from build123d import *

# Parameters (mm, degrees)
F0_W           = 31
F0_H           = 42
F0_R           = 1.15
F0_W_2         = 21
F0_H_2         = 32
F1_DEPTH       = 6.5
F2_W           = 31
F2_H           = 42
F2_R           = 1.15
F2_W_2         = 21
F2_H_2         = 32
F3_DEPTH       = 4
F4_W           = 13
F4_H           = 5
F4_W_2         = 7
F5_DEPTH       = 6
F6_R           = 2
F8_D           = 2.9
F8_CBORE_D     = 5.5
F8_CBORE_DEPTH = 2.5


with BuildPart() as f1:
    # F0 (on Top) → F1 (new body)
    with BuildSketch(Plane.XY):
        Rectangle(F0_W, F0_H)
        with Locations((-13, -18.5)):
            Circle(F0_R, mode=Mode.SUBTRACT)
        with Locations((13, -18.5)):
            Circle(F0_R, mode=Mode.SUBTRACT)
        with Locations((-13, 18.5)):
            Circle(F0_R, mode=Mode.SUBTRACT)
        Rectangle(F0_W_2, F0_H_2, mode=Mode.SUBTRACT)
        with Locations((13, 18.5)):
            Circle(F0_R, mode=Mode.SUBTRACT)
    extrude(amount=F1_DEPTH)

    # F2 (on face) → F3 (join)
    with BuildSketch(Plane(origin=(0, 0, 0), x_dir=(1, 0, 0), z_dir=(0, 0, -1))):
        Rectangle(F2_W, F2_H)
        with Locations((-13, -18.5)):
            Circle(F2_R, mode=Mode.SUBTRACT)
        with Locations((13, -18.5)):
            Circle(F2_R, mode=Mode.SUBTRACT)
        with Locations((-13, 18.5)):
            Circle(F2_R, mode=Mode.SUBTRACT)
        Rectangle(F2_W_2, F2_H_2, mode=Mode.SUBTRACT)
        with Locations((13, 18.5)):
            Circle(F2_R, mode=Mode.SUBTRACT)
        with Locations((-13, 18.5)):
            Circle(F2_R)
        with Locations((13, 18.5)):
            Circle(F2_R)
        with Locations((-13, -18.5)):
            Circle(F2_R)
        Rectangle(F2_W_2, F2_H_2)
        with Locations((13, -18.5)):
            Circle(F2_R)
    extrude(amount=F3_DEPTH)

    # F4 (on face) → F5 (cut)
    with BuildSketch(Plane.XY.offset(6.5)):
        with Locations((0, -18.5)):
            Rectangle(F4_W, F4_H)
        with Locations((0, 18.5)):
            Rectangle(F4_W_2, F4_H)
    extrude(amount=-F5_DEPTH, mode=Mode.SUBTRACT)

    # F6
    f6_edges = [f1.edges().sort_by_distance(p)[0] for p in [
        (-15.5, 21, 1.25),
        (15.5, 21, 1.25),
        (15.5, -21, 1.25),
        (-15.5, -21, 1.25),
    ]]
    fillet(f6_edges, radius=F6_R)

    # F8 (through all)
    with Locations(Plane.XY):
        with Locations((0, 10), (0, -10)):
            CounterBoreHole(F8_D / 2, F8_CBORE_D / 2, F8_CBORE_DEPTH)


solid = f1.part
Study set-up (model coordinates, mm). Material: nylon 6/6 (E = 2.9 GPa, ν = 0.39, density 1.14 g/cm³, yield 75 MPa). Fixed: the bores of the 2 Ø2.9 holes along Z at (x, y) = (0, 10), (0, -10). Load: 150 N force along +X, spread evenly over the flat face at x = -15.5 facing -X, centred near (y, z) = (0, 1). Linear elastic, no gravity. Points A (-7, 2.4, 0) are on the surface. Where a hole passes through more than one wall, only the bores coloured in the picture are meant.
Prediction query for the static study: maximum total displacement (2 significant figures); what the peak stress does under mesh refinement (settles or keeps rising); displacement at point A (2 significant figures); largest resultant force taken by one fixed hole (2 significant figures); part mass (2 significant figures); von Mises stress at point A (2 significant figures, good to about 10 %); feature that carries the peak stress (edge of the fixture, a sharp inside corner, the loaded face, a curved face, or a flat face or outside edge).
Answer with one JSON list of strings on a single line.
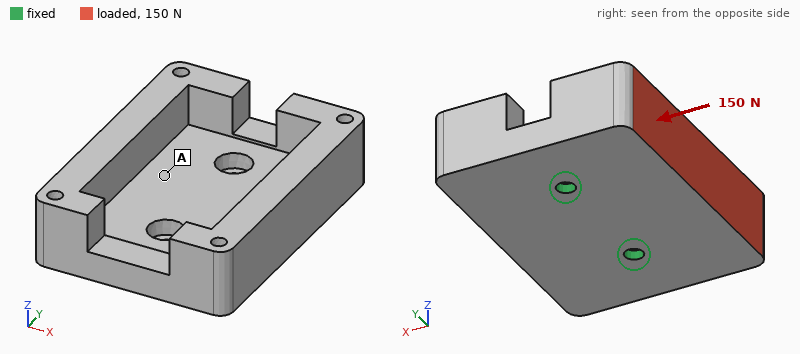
["0.42 mm", "keeps rising", "0.16 mm", "75 N", "9.6 g", "4.4 MPa", "edge of the fixture"]
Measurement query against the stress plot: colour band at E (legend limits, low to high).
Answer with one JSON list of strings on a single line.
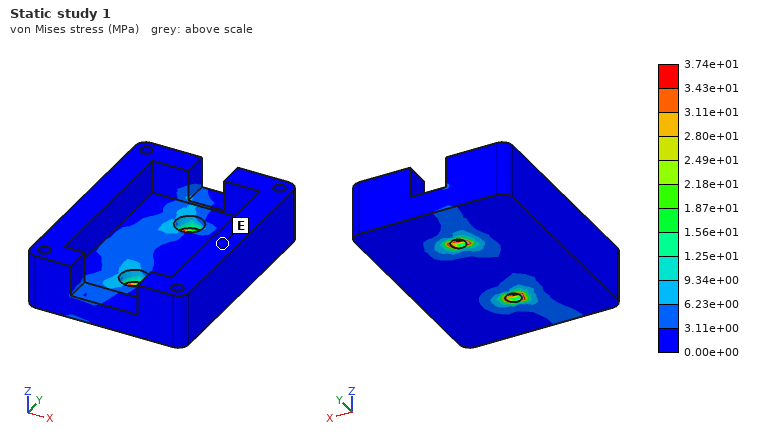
["0.00e+00 to 3.11e+00 MPa"]
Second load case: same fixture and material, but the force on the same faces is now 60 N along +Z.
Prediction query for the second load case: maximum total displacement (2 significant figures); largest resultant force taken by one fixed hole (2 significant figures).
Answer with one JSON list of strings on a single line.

["0.54 mm", "30 N"]
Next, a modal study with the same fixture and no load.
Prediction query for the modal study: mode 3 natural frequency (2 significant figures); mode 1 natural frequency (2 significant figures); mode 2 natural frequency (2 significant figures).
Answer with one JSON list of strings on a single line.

["2600 Hz", "880 Hz", "2500 Hz"]
